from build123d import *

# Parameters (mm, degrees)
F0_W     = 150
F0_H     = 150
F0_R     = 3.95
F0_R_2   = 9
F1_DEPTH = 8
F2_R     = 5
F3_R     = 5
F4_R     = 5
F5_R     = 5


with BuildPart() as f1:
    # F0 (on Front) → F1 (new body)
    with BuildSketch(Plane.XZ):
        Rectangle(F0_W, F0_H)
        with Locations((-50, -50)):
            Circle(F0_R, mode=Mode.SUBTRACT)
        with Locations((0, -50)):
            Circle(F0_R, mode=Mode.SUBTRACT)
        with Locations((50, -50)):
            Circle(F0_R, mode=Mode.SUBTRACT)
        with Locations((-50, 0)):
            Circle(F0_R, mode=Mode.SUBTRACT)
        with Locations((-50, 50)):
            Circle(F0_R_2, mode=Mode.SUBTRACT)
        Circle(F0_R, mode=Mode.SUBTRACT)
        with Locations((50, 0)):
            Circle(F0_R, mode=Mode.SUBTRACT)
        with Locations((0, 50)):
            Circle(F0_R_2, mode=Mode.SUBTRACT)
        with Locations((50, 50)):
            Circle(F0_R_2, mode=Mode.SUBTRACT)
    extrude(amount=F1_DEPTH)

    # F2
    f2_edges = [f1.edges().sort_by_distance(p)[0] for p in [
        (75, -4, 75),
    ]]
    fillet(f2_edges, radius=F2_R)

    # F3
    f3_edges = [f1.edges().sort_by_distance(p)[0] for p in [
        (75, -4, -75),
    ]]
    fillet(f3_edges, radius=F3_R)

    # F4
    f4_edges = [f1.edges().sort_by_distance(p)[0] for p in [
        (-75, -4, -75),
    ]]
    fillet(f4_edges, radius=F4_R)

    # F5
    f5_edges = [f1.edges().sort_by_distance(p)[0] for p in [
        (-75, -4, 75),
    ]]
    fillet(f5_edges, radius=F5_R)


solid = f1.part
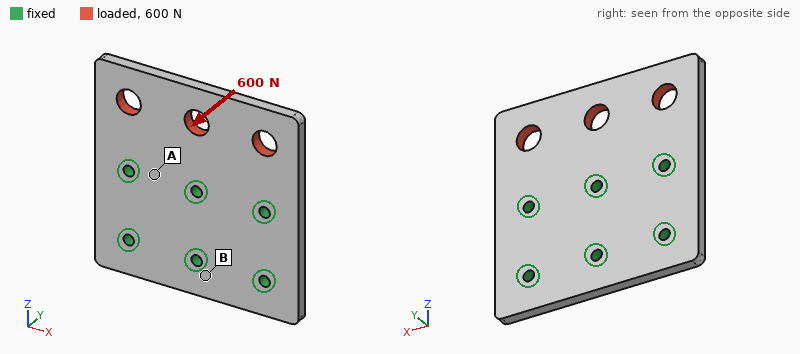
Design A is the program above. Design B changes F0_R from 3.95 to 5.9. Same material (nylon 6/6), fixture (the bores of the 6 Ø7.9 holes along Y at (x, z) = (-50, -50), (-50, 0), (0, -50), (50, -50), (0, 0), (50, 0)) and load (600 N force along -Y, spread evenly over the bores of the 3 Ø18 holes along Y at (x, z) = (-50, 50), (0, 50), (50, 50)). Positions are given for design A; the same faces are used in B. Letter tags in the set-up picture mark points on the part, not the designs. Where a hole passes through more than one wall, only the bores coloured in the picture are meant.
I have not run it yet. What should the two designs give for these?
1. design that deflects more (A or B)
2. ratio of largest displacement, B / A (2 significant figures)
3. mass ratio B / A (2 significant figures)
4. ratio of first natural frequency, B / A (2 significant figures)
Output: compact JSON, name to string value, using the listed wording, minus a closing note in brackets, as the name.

{"design that deflects more": "A", "ratio of largest displacement, B / A": "0.87", "mass ratio B / A": "0.98", "ratio of first natural frequency, B / A": "1.1"}
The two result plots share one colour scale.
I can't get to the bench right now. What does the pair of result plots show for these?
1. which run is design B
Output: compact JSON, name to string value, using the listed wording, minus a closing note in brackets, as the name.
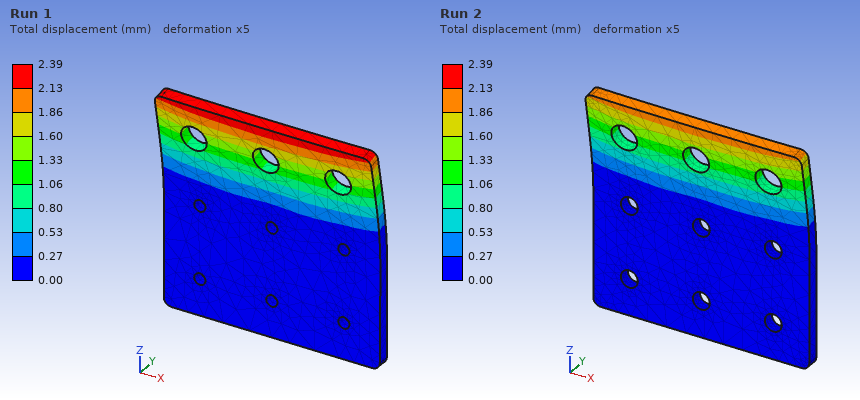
{"which run is design B": "Run 2"}
